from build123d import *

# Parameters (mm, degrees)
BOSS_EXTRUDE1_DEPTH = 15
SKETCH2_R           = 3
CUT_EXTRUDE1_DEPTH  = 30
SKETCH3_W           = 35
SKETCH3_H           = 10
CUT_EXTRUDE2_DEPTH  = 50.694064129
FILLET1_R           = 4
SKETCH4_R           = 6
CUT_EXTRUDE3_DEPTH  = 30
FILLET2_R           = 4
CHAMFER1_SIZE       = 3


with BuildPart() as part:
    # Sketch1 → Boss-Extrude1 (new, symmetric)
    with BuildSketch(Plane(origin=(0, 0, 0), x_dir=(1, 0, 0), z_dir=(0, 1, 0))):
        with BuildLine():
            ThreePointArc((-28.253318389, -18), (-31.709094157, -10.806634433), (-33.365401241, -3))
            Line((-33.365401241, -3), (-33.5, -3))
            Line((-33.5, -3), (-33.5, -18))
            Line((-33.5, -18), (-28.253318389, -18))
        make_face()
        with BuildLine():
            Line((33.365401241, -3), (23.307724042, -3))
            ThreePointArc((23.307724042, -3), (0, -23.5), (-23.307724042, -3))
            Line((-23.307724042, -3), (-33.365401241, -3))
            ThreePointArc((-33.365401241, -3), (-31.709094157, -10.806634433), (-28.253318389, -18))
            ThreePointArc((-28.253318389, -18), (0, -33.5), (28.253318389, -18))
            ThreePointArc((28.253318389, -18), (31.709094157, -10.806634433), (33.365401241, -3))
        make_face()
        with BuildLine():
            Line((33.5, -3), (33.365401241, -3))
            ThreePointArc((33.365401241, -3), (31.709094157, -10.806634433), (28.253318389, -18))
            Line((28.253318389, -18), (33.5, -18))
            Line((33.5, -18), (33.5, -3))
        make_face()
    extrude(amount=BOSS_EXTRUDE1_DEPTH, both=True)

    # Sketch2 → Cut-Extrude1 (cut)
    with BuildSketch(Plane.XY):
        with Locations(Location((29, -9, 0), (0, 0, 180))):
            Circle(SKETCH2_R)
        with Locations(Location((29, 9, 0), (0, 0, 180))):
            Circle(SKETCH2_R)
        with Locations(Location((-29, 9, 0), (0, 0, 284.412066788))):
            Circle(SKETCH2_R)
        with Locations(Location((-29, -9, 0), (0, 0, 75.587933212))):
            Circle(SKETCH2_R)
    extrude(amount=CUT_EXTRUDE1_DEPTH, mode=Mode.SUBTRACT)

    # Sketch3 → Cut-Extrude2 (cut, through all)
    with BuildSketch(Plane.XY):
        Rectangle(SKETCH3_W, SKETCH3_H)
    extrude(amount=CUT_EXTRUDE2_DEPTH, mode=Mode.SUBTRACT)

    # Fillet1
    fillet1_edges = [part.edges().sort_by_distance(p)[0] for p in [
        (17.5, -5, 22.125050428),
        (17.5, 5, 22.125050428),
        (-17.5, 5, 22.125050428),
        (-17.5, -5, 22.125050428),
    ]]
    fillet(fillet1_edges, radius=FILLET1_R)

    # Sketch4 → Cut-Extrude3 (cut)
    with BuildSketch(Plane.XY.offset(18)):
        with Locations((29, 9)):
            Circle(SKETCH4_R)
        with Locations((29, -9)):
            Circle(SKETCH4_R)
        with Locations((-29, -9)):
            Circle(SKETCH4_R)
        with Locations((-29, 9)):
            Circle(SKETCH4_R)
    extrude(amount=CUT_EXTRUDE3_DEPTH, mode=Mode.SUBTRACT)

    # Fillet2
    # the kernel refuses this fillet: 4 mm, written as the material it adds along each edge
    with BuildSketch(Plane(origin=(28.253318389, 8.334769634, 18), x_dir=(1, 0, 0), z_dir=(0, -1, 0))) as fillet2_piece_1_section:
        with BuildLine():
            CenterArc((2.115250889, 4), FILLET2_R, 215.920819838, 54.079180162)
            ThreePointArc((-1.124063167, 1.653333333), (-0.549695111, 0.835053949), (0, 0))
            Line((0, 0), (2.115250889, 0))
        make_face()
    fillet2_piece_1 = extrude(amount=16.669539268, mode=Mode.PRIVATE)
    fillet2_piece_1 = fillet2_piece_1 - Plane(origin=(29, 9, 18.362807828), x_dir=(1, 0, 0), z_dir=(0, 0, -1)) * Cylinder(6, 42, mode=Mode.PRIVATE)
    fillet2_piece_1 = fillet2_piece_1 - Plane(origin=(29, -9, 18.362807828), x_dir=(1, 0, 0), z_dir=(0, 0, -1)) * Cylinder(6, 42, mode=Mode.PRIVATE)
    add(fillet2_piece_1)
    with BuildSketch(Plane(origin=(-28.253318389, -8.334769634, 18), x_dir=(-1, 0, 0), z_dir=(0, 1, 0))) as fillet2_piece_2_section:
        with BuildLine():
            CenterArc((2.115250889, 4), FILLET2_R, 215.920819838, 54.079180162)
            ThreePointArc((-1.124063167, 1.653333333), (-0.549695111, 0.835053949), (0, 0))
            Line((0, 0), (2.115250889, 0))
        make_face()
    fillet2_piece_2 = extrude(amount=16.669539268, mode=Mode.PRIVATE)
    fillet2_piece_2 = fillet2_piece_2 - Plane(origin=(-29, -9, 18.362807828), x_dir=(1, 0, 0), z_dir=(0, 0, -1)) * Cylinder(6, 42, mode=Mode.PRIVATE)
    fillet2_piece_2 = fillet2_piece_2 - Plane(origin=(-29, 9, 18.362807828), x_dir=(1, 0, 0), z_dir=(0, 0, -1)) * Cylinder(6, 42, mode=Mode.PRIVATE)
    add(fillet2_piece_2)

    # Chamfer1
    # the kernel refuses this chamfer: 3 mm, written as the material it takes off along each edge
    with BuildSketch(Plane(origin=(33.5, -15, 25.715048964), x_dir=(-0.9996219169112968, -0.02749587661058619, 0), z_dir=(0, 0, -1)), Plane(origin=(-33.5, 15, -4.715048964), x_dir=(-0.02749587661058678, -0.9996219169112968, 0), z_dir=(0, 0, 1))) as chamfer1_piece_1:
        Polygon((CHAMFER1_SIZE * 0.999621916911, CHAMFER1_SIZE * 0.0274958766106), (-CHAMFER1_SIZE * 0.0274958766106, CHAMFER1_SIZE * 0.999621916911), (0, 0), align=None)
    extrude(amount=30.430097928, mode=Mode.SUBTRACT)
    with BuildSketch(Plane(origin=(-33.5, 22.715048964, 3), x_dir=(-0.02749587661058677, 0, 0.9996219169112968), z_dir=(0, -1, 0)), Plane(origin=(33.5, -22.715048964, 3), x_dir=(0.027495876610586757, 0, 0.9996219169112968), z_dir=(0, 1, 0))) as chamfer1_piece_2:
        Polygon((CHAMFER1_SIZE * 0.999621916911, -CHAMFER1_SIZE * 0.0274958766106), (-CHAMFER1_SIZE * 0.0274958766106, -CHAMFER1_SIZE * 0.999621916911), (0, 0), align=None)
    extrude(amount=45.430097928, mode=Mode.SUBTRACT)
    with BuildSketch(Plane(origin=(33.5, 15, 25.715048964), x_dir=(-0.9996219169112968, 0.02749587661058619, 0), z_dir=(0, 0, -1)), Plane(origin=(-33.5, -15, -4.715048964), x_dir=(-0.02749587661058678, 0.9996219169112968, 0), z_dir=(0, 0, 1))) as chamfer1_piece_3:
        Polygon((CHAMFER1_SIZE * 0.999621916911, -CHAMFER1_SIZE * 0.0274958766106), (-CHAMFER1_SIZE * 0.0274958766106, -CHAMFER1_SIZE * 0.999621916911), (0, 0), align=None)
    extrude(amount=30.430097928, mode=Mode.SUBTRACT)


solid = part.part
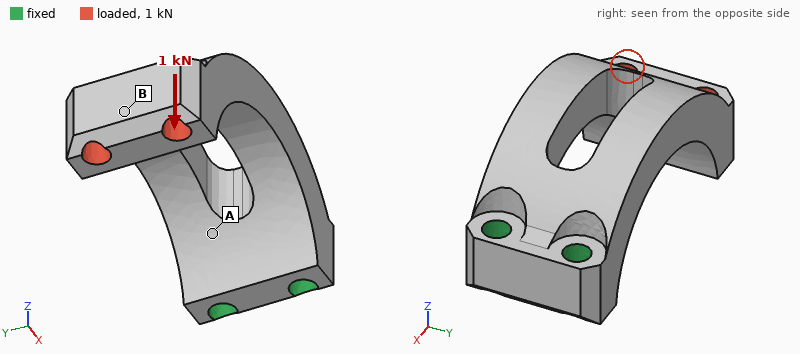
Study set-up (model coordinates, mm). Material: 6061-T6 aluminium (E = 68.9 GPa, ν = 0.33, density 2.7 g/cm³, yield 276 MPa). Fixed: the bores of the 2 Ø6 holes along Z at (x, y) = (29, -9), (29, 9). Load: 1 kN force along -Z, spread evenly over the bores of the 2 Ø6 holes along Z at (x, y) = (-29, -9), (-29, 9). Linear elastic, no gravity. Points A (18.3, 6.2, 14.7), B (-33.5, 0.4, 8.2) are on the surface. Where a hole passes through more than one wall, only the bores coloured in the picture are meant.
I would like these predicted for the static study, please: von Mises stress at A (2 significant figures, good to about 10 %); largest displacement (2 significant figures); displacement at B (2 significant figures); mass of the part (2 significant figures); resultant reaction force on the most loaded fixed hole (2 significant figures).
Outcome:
160 MPa
0.76 mm
0.75 mm
55 g
550 N
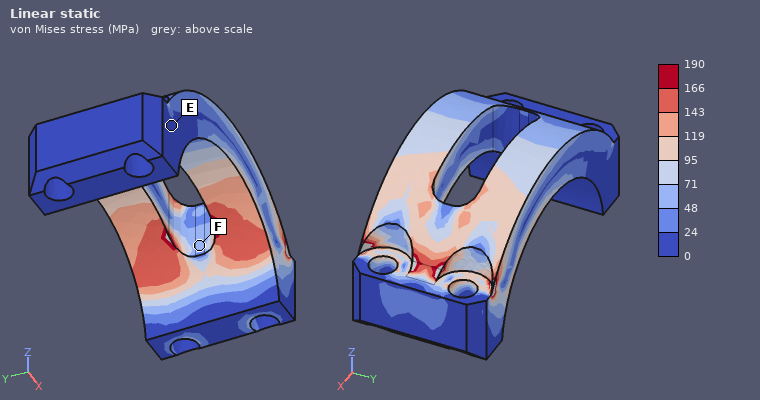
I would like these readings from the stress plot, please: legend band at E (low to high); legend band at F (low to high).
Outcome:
0 to 24 MPa
48 to 71 MPa
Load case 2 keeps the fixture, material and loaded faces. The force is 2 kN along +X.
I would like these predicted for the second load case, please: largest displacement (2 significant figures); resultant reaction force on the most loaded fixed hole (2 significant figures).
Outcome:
0.52 mm
1.0 kN
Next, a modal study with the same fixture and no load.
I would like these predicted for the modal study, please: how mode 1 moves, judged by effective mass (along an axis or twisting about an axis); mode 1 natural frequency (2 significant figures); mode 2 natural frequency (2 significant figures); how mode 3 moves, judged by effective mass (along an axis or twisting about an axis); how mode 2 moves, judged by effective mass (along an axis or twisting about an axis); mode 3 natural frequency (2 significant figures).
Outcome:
along Z
1500 Hz
2000 Hz
along X
along Y
5300 Hz
